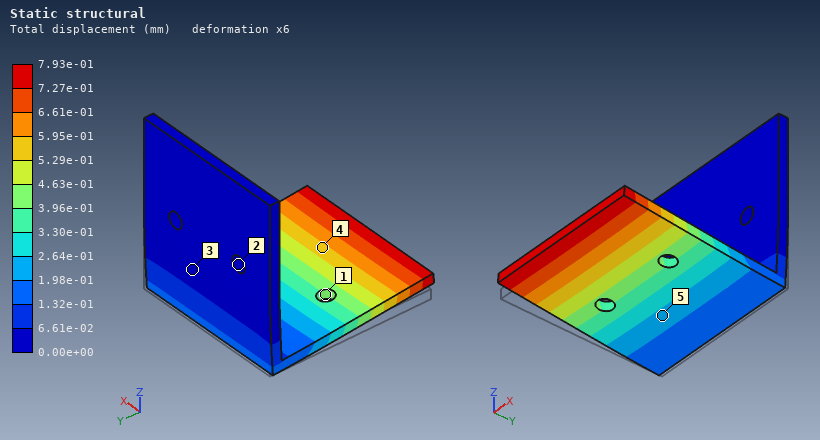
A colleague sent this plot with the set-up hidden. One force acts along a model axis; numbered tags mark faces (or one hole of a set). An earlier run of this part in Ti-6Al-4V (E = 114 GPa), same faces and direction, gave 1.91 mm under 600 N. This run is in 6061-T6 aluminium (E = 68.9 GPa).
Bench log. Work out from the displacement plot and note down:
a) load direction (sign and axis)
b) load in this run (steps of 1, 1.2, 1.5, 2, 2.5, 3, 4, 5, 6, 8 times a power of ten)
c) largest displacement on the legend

+Z
150 N
7.93e-01 mm
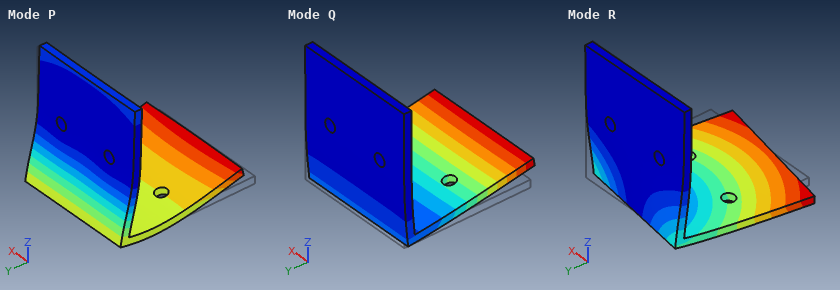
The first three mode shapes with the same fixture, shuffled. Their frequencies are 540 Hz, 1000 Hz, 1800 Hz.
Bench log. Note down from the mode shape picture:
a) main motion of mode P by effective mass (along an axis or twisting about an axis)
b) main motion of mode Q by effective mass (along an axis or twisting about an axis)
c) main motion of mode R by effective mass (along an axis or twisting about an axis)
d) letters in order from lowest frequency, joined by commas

along Y
along Z
along X
Q, R, P
